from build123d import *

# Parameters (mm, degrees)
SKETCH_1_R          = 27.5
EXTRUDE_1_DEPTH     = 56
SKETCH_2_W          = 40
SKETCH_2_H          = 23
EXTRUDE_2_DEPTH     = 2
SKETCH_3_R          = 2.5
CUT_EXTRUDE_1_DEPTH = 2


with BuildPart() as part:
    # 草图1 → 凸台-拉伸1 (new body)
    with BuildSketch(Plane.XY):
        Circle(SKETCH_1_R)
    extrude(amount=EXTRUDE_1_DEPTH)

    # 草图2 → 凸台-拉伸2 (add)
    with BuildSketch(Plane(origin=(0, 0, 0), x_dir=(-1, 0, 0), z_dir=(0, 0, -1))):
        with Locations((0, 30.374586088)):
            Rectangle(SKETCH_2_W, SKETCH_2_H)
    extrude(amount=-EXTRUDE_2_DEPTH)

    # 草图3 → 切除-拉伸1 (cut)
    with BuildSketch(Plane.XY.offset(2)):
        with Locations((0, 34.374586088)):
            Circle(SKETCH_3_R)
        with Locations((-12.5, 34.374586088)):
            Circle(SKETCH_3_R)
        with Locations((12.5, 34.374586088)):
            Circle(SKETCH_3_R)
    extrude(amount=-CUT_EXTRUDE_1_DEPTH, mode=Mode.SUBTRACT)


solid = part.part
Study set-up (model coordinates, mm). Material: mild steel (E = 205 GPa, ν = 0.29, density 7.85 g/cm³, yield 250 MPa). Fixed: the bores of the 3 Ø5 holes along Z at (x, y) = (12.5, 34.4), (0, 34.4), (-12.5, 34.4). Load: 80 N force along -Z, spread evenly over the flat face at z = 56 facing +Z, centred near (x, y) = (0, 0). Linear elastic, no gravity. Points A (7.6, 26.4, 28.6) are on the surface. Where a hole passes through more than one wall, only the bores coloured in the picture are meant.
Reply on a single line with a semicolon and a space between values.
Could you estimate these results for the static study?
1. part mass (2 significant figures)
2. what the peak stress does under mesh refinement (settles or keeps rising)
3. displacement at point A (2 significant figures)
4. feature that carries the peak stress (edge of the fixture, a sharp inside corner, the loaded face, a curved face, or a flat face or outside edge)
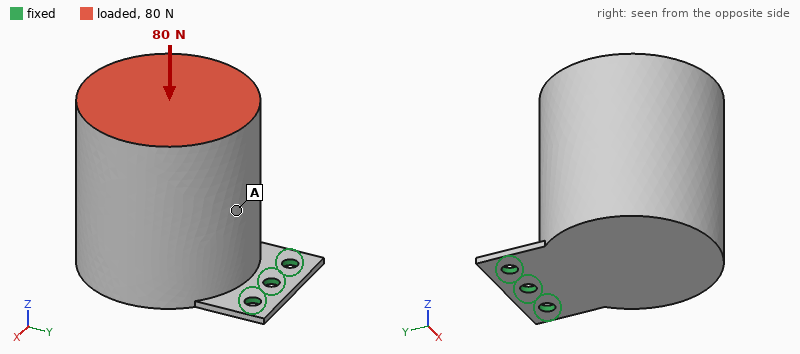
1.1 kg; keeps rising; 0.083 mm; edge of the fixture
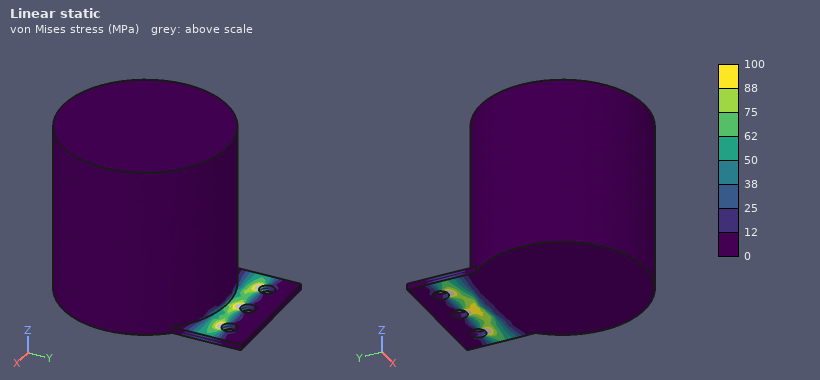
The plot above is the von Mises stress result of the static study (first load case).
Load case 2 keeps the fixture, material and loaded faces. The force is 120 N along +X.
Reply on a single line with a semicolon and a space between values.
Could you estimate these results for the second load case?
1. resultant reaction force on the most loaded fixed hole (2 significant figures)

300 N
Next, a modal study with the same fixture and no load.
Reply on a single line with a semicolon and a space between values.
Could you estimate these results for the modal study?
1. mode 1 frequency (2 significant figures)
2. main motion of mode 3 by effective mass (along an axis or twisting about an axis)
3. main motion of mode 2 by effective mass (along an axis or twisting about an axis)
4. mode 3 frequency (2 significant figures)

96 Hz; along X; along X; 2000 Hz
